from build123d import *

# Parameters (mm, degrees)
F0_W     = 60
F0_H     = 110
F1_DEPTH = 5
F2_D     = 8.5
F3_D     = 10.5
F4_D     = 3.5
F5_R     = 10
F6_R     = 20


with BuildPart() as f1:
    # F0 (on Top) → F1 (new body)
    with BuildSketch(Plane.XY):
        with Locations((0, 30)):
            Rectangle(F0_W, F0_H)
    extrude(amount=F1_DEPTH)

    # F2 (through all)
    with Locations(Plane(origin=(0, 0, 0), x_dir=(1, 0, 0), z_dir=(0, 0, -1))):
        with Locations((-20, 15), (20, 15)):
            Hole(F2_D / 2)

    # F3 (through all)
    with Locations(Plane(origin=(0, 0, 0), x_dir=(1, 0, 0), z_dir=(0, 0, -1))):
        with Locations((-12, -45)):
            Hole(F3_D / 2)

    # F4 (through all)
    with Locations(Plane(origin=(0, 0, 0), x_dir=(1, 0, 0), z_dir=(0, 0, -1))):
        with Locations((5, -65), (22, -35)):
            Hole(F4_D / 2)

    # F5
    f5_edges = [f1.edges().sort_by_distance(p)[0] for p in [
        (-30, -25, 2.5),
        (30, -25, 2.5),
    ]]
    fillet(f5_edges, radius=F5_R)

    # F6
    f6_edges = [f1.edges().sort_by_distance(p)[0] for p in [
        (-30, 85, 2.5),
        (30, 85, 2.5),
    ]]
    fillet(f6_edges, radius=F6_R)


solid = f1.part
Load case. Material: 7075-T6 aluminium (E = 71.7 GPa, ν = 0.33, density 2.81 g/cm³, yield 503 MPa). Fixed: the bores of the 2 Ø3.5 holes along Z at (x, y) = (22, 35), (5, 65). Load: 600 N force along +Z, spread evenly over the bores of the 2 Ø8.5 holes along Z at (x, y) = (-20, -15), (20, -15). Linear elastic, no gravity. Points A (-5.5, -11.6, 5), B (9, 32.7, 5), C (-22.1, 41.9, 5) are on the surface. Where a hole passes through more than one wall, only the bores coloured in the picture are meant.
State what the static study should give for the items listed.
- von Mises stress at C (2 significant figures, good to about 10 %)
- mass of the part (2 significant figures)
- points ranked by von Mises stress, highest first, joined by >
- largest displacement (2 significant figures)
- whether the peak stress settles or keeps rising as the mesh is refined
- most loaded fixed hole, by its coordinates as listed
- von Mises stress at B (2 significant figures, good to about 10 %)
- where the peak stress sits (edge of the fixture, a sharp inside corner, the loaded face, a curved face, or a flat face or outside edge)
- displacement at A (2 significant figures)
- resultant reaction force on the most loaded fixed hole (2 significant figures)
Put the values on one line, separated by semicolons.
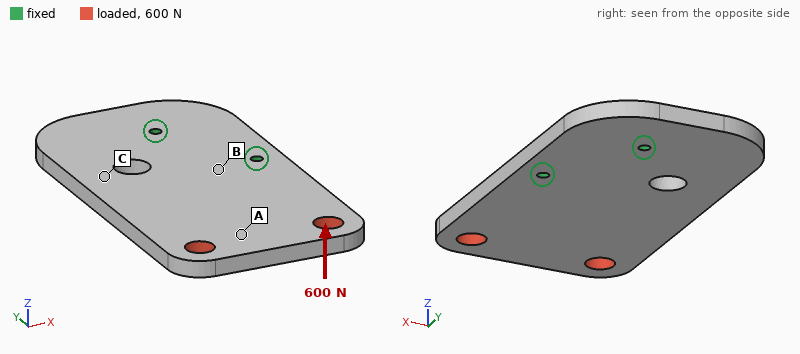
74 MPa; 87 g; B > C > A; 1.4 mm; keeps rising; (22, 35); 120 MPa; edge of the fixture; 0.96 mm; 970 N
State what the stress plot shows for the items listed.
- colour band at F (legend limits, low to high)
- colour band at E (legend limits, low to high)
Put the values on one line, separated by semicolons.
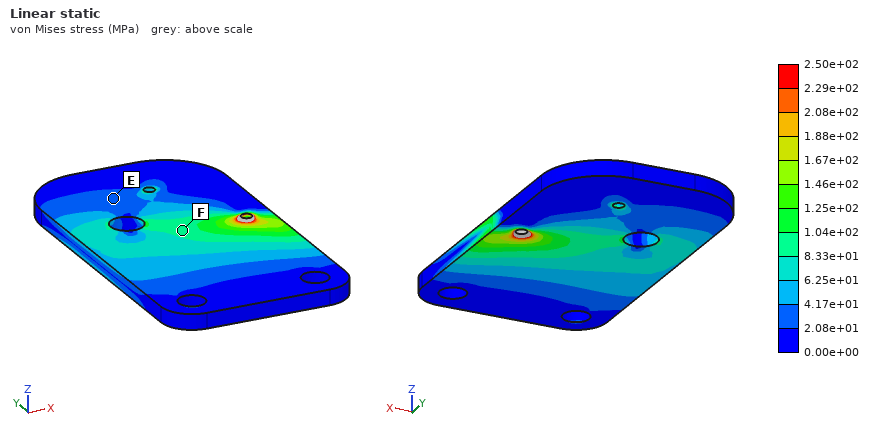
8.33e+01 to 1.04e+02 MPa; 2.08e+01 to 4.17e+01 MPa
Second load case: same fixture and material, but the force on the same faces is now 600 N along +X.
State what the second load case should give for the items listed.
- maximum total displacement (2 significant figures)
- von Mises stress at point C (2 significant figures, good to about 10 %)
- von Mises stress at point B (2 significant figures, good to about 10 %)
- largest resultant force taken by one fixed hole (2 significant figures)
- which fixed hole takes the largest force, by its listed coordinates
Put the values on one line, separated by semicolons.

27 µm; 7.4 MPa; 8.8 MPa; 1.3 kN; (22, 35)
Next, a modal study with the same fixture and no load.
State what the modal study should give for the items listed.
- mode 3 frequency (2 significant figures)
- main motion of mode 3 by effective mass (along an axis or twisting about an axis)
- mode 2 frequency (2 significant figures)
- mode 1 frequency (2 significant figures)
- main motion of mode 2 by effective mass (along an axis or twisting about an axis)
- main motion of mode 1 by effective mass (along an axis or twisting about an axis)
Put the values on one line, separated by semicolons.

3300 Hz; along Z; 1800 Hz; 810 Hz; twisting about Y; along Z
